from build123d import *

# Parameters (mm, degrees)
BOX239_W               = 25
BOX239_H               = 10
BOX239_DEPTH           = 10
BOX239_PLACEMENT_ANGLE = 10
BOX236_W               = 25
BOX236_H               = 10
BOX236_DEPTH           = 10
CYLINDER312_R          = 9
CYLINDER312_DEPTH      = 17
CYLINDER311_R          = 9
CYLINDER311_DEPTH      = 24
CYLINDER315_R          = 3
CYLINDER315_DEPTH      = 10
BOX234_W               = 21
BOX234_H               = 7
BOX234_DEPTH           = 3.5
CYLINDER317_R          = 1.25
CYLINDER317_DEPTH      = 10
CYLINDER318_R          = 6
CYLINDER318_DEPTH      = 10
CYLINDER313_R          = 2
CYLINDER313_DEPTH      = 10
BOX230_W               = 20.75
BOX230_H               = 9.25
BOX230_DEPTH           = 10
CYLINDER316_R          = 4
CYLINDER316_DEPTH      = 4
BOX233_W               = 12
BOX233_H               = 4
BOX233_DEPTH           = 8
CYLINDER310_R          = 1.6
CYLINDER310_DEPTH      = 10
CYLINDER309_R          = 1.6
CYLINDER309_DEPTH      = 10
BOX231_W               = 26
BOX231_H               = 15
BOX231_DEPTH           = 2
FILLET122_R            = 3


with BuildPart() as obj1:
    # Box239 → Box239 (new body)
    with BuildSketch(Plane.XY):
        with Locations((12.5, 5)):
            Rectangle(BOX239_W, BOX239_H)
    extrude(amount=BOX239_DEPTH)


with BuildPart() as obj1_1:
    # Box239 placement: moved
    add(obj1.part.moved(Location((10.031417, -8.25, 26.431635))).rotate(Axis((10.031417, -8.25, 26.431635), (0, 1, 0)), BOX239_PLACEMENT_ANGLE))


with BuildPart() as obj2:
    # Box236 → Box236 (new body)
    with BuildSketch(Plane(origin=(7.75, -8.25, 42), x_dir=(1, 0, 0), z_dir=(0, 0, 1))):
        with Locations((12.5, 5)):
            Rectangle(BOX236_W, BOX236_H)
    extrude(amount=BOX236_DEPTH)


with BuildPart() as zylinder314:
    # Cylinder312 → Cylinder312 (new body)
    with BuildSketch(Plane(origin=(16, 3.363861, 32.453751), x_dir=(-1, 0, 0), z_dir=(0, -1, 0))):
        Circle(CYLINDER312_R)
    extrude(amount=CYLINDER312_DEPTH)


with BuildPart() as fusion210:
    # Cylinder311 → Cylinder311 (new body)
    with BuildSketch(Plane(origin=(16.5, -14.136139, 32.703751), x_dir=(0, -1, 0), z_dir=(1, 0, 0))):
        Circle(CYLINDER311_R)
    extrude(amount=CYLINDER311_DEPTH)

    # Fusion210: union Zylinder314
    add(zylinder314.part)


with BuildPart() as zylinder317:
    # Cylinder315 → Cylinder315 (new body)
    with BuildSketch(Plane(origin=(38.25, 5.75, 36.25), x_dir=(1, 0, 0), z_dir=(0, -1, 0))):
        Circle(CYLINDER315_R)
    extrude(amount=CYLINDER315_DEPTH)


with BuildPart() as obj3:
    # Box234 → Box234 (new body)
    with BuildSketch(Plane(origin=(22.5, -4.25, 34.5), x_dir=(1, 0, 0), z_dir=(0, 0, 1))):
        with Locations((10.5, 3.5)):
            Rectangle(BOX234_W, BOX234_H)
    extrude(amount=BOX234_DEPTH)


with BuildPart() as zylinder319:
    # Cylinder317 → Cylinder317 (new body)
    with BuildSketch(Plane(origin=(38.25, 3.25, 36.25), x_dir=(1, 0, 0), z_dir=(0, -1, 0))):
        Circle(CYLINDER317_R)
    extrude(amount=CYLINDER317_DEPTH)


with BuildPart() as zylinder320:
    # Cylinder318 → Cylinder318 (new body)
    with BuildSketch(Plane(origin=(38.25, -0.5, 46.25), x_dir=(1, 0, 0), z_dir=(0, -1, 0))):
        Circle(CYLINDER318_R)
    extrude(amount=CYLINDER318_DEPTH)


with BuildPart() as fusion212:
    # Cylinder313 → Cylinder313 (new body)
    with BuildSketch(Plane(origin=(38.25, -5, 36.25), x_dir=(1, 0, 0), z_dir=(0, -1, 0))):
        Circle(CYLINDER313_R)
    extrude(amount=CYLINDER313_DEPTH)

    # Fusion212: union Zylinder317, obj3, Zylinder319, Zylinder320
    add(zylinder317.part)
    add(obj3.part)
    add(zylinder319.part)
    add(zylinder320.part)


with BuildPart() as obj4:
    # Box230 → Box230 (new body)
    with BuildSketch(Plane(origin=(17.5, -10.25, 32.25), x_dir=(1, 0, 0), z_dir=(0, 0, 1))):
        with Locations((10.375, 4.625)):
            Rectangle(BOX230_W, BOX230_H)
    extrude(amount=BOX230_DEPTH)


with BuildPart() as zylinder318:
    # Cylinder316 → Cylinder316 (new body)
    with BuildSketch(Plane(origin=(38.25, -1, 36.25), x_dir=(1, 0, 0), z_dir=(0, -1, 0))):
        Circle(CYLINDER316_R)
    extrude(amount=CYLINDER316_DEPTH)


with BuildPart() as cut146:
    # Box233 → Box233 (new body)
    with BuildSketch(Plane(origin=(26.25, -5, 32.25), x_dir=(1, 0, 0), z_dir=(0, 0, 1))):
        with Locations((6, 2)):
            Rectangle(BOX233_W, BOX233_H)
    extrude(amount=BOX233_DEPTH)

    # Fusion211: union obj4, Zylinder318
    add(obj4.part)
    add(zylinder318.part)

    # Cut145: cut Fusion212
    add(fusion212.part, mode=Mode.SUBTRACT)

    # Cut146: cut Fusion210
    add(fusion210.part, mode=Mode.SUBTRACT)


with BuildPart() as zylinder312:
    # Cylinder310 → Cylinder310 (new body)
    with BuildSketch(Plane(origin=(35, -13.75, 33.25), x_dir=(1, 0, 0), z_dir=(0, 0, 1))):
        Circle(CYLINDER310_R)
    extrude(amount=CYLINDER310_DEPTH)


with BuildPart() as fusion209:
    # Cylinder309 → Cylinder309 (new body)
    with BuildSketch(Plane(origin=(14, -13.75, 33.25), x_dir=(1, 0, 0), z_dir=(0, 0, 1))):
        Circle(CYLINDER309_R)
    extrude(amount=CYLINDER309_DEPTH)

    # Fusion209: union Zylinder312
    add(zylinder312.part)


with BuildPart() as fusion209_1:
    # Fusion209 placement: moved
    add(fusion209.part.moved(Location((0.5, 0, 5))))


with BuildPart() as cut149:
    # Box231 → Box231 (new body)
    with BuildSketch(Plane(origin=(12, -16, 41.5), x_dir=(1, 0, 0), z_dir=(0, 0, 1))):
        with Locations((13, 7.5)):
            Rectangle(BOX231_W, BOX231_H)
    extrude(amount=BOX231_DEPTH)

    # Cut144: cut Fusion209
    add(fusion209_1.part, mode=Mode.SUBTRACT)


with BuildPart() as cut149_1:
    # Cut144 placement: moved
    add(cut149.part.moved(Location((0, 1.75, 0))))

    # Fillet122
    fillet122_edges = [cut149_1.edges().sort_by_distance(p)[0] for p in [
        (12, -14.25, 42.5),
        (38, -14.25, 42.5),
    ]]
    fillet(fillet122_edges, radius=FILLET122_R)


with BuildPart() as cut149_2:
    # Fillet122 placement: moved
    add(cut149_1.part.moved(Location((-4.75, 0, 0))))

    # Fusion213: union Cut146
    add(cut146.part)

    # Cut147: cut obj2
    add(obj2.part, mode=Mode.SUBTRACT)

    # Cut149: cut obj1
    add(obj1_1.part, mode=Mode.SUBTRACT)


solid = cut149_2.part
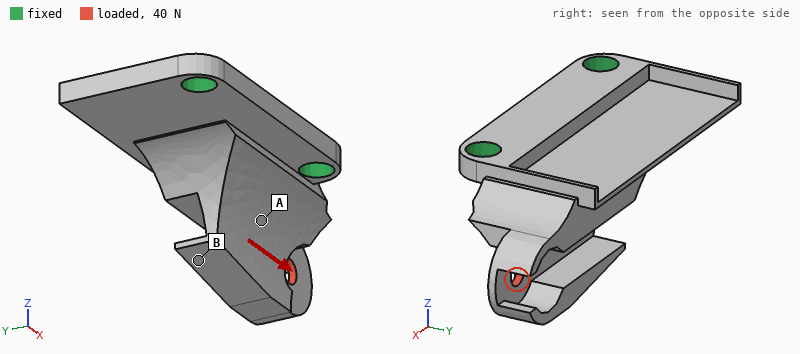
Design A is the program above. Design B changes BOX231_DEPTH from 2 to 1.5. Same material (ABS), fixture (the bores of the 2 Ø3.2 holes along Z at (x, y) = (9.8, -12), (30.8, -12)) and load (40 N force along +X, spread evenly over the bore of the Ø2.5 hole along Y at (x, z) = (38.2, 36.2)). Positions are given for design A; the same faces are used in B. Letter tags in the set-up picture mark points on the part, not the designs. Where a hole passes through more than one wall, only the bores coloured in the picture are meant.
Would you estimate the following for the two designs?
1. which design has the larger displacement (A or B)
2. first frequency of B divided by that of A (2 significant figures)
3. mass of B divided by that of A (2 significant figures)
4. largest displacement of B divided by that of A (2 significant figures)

B
0.79
0.93
1.4
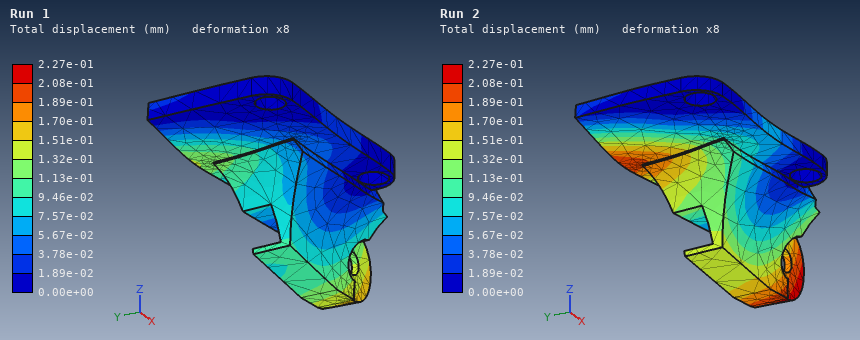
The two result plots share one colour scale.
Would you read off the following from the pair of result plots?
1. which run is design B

Run 2
